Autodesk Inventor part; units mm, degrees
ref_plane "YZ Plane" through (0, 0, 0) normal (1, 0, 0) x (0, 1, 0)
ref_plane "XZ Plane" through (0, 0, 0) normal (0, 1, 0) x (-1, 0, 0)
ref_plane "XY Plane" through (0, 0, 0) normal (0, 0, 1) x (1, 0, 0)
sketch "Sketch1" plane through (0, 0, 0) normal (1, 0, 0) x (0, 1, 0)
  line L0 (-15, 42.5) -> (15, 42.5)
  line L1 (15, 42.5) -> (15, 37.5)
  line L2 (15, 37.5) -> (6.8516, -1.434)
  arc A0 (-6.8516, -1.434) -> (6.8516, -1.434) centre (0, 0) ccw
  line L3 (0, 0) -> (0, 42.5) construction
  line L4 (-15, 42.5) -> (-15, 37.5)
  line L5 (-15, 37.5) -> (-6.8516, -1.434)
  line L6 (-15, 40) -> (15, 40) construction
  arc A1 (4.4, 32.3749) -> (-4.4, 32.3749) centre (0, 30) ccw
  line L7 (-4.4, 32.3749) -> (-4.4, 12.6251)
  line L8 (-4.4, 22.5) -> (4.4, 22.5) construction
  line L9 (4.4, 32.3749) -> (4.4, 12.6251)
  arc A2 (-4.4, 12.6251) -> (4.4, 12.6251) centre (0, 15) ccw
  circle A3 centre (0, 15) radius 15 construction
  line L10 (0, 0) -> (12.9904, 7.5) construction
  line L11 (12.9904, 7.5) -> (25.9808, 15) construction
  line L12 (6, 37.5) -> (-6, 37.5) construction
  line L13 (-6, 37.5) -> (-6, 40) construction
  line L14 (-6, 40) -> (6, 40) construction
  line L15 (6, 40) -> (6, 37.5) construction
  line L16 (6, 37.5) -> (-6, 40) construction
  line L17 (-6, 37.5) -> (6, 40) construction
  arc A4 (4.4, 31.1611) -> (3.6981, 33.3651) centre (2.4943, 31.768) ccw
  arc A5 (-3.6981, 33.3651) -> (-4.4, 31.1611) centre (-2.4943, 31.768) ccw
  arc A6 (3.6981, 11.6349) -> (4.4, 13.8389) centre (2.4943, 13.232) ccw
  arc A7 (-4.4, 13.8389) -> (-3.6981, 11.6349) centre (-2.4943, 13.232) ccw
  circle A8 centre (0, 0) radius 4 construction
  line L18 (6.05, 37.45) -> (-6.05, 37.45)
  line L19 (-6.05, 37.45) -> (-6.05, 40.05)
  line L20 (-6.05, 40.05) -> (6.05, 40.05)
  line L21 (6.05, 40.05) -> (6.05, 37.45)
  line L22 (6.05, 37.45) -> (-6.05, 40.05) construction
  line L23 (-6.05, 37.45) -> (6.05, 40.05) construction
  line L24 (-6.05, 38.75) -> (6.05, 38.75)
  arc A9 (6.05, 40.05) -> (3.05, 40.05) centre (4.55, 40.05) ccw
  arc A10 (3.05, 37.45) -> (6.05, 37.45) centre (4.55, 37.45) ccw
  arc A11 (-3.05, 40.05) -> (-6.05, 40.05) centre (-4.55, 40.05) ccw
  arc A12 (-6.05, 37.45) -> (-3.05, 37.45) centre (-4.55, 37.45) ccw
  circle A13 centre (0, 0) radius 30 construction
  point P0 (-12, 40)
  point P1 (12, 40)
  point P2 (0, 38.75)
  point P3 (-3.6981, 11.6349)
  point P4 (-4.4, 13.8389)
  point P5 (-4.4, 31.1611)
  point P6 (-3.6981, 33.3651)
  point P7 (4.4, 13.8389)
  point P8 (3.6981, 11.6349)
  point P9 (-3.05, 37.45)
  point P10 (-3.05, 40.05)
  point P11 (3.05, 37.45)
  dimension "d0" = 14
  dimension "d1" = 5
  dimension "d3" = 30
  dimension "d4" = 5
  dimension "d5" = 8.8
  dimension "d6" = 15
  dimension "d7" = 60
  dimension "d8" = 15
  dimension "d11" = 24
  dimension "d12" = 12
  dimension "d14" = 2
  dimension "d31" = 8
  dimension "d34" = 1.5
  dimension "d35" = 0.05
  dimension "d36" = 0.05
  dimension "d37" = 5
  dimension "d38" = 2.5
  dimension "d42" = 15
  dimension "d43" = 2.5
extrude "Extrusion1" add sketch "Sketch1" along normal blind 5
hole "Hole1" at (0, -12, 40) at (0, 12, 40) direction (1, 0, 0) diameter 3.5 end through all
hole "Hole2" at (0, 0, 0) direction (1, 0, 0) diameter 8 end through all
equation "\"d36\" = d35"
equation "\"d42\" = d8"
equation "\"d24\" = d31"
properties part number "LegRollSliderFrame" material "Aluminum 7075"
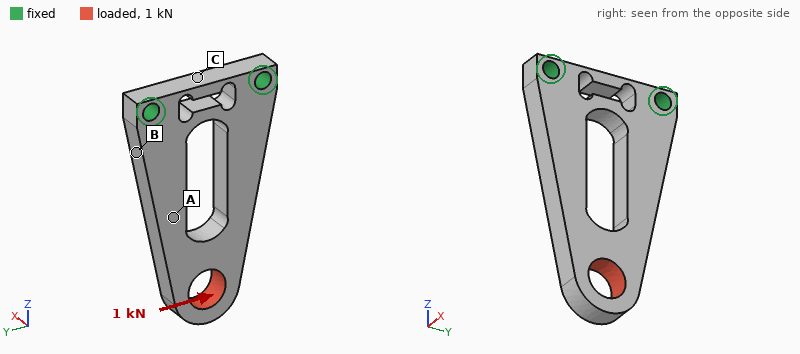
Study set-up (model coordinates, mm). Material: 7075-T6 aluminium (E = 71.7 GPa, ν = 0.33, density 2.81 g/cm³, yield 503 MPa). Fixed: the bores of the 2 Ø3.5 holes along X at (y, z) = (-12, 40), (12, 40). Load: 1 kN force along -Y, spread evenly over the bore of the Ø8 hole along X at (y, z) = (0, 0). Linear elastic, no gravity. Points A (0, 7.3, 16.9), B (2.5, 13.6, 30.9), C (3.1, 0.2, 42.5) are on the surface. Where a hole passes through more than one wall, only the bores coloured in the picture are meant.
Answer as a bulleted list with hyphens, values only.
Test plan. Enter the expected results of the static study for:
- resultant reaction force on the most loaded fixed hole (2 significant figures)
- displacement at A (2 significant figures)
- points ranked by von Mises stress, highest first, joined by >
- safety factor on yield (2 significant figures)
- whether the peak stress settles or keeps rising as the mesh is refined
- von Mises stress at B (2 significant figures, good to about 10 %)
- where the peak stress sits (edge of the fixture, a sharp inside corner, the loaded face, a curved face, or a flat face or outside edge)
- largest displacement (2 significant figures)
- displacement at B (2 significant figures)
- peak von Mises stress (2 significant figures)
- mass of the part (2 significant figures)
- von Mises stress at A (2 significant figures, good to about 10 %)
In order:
- 1.4 kN
- 0.069 mm
- B > A > C
- 2.1
- settles
- 93 MPa
- a curved face
- 0.12 mm
- 0.018 mm
- 240 MPa
- 10 g
- 56 MPa
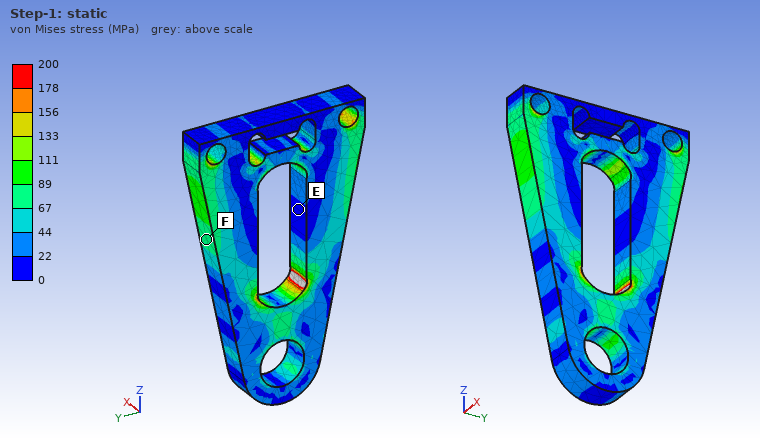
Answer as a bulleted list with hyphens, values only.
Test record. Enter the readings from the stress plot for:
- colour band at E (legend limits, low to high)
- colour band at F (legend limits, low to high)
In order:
- 0 to 22 MPa
- 67 to 89 MPa
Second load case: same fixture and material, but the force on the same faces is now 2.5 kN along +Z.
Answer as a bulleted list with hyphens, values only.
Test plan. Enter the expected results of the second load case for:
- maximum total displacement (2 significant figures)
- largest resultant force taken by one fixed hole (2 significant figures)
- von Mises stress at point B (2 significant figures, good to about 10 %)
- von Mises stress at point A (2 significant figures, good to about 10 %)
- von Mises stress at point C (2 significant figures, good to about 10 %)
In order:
- 28 µm
- 1.3 kN
- 37 MPa
- 42 MPa
- 7.7 MPa
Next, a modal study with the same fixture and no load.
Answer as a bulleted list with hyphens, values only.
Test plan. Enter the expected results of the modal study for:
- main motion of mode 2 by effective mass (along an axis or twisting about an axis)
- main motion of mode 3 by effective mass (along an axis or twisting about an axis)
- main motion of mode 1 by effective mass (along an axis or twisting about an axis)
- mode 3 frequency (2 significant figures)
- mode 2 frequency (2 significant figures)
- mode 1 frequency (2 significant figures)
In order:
- along Y
- twisting about Z
- along X
- 9100 Hz
- 7600 Hz
- 2400 Hz
